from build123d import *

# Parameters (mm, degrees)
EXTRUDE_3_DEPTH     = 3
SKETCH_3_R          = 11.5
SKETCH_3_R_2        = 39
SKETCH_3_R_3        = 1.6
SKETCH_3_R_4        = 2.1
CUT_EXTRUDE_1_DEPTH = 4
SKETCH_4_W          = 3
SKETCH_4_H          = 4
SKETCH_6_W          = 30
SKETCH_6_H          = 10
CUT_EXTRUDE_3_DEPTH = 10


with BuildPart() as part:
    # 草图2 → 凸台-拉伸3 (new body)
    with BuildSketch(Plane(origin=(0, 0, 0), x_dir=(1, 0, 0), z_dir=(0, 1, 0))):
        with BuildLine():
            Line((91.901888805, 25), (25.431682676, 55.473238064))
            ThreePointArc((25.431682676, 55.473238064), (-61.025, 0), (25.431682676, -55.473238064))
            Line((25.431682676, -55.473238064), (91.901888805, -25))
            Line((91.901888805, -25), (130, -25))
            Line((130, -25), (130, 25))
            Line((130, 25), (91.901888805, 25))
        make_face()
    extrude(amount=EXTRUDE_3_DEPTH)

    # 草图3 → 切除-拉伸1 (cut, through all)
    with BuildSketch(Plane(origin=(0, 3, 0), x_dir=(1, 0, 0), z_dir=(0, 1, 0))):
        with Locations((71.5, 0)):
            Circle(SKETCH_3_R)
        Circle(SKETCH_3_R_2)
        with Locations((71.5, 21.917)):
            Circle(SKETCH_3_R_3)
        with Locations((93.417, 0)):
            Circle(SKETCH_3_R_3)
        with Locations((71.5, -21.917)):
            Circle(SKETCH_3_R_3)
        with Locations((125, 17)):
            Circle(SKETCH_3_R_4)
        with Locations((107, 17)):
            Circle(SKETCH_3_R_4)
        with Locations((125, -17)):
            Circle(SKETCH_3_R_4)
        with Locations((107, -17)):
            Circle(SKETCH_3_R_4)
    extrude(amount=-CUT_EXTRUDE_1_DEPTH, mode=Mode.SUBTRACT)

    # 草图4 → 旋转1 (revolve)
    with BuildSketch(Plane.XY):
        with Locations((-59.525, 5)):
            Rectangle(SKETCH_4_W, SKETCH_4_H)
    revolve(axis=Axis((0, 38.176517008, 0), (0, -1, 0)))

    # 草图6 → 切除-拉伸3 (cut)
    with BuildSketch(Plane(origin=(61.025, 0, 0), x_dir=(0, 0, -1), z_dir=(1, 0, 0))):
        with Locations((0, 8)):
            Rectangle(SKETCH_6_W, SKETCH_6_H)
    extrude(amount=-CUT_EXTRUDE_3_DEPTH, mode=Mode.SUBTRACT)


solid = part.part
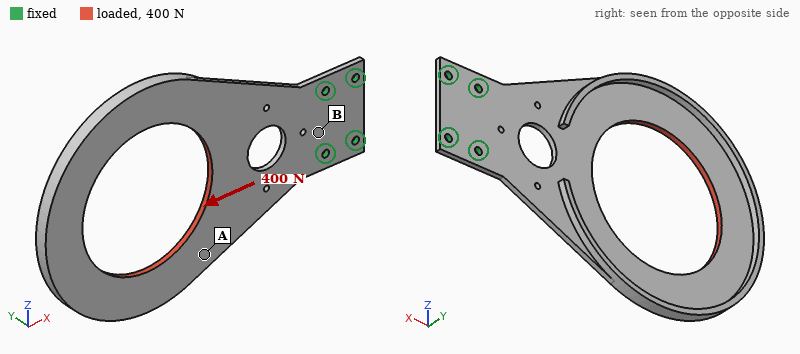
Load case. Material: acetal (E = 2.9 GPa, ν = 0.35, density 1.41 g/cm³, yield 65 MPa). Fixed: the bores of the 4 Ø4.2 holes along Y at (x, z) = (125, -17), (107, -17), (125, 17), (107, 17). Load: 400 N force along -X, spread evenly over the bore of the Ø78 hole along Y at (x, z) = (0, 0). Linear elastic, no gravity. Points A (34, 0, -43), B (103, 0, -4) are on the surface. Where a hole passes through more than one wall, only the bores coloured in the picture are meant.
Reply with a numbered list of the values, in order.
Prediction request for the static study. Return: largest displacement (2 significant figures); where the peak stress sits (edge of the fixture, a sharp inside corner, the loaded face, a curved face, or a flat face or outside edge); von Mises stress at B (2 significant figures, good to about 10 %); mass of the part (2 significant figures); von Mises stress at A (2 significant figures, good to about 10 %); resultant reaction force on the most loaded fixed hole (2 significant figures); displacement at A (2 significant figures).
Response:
1. 0.32 mm
2. a curved face
3. 1.2 MPa
4. 52 g
5. 3.0 MPa
6. 160 N
7. 0.14 mm
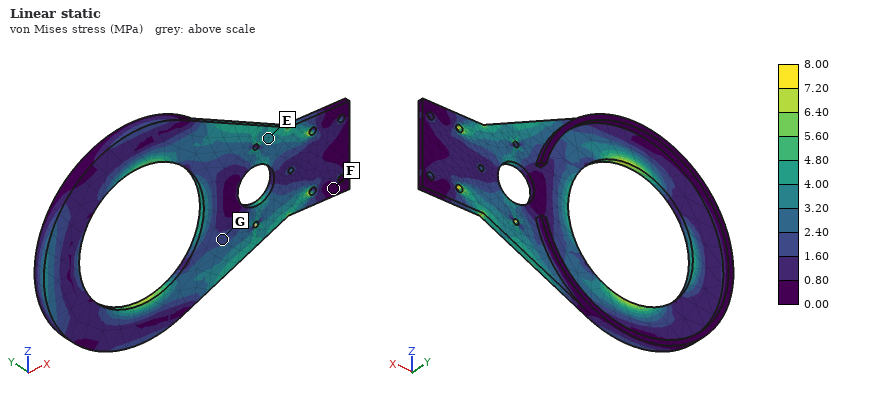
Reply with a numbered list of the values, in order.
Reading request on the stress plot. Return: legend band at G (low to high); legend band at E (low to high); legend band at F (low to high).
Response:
1. 1.60 to 2.40 MPa
2. 3.20 to 4.00 MPa
3. 0.00 to 0.80 MPa
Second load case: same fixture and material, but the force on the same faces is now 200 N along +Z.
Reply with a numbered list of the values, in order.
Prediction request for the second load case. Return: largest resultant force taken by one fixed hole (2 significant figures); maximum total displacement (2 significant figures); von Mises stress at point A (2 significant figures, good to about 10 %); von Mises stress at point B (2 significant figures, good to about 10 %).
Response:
1. 520 N
2. 2.4 mm
3. 3.6 MPa
4. 3.3 MPa
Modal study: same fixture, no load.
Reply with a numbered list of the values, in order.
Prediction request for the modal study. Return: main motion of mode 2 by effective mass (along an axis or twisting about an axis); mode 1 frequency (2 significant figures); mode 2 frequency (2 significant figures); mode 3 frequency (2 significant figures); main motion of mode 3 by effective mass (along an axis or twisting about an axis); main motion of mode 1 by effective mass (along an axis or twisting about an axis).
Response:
1. twisting about X
2. 21 Hz
3. 65 Hz
4. 160 Hz
5. along Y
6. along Y
